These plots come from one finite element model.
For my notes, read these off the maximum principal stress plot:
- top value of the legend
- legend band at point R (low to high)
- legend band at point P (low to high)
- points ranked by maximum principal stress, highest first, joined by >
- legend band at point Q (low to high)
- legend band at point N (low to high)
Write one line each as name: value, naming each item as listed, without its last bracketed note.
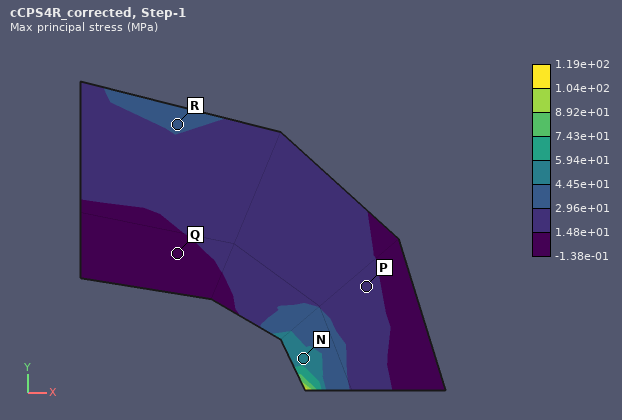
top value of the legend: 1.19e+02 MPa
legend band at point R: 2.96e+01 to 4.45e+01 MPa
legend band at point P: 1.48e+01 to 2.96e+01 MPa
points ranked by maximum principal stress, highest first, joined by >: N > R > P > Q
legend band at point Q: -1.38e-01 to 1.48e+01 MPa
legend band at point N: 4.45e+01 to 5.94e+01 MPa
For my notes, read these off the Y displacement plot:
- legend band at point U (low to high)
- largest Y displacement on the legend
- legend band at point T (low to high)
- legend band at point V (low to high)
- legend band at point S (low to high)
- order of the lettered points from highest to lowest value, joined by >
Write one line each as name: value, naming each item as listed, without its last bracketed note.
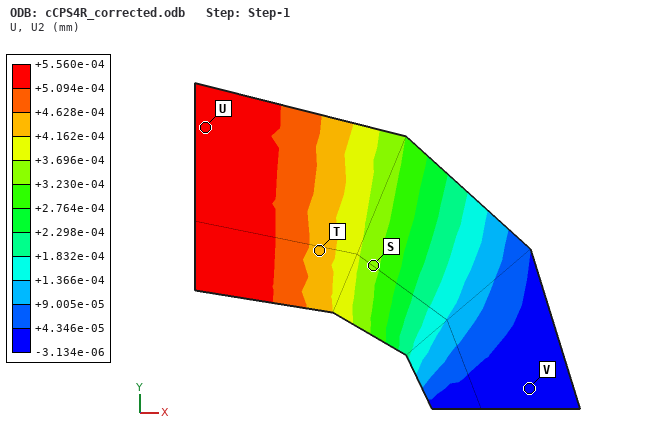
legend band at point U: +5.094e-04 to +5.560e-04 mm
largest Y displacement on the legend: +5.560e-04 mm
legend band at point T: +4.162e-04 to +4.628e-04 mm
legend band at point V: -3.134e-06 to +4.346e-05 mm
legend band at point S: +3.230e-04 to +3.696e-04 mm
order of the lettered points from highest to lowest value, joined by >: U > T > S > V
